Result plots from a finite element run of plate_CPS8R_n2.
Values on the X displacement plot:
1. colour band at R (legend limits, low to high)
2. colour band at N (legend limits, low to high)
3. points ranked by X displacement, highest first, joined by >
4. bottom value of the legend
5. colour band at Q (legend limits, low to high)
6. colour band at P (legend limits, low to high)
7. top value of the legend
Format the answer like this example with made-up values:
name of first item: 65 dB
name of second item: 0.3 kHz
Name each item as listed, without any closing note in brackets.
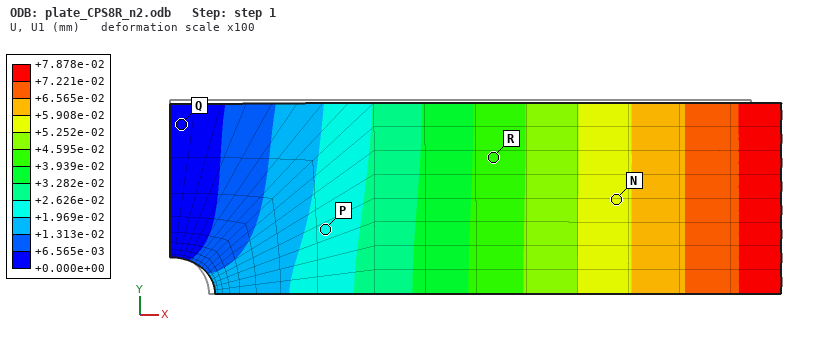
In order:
colour band at R: +3.939e-02 to +4.595e-02 mm
colour band at N: +5.252e-02 to +5.908e-02 mm
points ranked by X displacement, highest first, joined by >: N > R > P > Q
bottom value of the legend: +0.000e+00 mm
colour band at Q: +0.000e+00 to +6.565e-03 mm
colour band at P: +1.969e-02 to +2.626e-02 mm
top value of the legend: +7.878e-02 mm
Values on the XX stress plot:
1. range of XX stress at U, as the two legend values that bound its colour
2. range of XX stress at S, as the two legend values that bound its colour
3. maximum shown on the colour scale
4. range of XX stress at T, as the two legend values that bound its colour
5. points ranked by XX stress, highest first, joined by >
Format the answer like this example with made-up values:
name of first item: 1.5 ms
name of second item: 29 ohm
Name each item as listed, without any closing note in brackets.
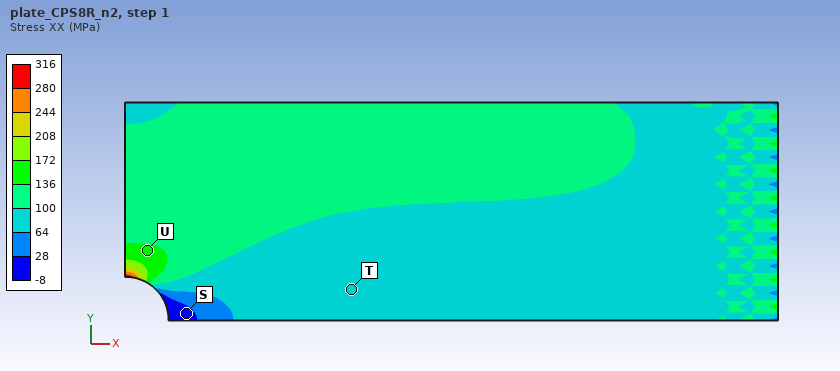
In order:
range of XX stress at U, as the two legend values that bound its colour: 136 to 172 MPa
range of XX stress at S, as the two legend values that bound its colour: -8 to 28 MPa
maximum shown on the colour scale: 316 MPa
range of XX stress at T, as the two legend values that bound its colour: 64 to 100 MPa
points ranked by XX stress, highest first, joined by >: U > T > S
